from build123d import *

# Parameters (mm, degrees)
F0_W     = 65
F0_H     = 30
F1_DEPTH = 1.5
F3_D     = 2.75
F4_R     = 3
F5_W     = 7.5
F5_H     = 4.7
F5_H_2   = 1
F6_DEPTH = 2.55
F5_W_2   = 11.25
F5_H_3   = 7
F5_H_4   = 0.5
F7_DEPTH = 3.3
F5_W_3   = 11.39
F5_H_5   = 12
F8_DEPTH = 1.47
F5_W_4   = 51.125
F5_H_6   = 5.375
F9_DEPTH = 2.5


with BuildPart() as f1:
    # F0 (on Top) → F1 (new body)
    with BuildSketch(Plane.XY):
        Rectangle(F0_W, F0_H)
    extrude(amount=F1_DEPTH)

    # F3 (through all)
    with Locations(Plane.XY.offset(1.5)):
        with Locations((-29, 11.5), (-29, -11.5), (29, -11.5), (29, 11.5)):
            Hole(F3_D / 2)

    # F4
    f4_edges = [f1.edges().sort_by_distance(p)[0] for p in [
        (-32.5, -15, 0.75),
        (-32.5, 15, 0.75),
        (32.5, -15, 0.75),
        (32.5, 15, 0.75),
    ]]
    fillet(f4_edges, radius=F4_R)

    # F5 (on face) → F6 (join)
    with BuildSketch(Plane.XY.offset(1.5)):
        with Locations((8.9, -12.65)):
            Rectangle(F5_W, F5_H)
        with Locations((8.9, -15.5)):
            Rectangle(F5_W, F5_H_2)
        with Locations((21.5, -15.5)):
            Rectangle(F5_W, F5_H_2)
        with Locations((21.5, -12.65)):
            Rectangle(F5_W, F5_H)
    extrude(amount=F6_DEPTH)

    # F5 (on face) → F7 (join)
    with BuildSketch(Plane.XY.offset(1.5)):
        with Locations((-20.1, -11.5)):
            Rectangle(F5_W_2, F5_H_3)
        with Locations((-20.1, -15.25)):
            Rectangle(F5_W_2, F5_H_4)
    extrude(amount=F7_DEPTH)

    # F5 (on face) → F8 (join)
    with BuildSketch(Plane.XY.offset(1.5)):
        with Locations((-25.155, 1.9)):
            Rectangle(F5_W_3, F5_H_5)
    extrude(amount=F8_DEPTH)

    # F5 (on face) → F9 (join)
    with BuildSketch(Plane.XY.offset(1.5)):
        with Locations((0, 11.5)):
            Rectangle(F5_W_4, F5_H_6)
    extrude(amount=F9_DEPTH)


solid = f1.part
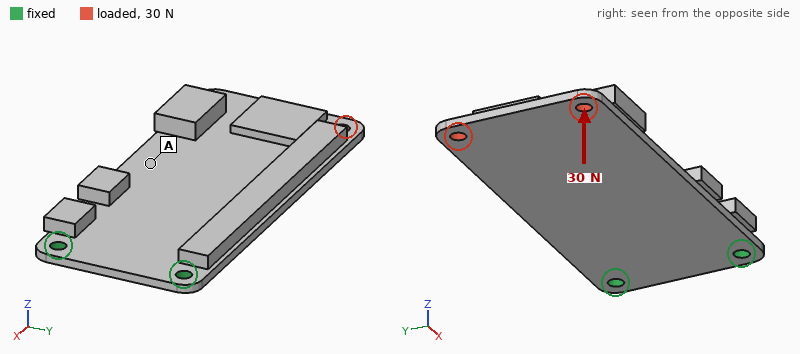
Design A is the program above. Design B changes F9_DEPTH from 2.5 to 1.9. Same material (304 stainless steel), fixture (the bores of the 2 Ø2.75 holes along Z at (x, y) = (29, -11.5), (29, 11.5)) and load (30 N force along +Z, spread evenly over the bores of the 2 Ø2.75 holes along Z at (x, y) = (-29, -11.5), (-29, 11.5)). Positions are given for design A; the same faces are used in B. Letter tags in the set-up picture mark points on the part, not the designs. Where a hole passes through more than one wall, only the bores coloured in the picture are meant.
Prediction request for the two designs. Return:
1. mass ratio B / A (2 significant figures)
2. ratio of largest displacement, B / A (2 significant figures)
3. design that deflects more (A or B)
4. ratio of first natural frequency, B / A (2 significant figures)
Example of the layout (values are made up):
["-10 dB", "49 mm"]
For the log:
["0.96", "1.1", "B", "0.97"]
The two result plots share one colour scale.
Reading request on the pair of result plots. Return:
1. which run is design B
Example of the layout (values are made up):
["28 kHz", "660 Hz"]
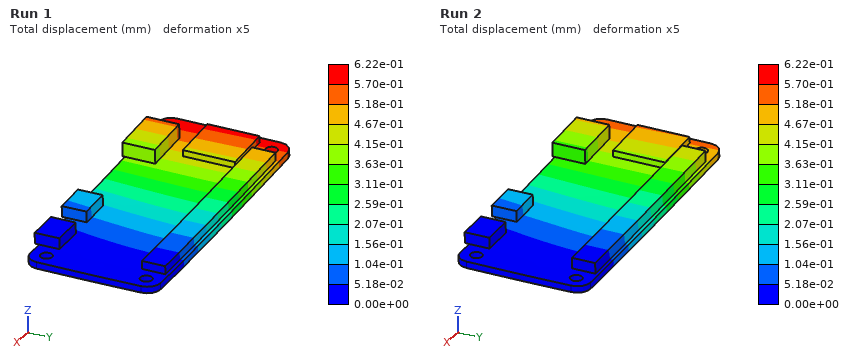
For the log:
["Run 1"]
